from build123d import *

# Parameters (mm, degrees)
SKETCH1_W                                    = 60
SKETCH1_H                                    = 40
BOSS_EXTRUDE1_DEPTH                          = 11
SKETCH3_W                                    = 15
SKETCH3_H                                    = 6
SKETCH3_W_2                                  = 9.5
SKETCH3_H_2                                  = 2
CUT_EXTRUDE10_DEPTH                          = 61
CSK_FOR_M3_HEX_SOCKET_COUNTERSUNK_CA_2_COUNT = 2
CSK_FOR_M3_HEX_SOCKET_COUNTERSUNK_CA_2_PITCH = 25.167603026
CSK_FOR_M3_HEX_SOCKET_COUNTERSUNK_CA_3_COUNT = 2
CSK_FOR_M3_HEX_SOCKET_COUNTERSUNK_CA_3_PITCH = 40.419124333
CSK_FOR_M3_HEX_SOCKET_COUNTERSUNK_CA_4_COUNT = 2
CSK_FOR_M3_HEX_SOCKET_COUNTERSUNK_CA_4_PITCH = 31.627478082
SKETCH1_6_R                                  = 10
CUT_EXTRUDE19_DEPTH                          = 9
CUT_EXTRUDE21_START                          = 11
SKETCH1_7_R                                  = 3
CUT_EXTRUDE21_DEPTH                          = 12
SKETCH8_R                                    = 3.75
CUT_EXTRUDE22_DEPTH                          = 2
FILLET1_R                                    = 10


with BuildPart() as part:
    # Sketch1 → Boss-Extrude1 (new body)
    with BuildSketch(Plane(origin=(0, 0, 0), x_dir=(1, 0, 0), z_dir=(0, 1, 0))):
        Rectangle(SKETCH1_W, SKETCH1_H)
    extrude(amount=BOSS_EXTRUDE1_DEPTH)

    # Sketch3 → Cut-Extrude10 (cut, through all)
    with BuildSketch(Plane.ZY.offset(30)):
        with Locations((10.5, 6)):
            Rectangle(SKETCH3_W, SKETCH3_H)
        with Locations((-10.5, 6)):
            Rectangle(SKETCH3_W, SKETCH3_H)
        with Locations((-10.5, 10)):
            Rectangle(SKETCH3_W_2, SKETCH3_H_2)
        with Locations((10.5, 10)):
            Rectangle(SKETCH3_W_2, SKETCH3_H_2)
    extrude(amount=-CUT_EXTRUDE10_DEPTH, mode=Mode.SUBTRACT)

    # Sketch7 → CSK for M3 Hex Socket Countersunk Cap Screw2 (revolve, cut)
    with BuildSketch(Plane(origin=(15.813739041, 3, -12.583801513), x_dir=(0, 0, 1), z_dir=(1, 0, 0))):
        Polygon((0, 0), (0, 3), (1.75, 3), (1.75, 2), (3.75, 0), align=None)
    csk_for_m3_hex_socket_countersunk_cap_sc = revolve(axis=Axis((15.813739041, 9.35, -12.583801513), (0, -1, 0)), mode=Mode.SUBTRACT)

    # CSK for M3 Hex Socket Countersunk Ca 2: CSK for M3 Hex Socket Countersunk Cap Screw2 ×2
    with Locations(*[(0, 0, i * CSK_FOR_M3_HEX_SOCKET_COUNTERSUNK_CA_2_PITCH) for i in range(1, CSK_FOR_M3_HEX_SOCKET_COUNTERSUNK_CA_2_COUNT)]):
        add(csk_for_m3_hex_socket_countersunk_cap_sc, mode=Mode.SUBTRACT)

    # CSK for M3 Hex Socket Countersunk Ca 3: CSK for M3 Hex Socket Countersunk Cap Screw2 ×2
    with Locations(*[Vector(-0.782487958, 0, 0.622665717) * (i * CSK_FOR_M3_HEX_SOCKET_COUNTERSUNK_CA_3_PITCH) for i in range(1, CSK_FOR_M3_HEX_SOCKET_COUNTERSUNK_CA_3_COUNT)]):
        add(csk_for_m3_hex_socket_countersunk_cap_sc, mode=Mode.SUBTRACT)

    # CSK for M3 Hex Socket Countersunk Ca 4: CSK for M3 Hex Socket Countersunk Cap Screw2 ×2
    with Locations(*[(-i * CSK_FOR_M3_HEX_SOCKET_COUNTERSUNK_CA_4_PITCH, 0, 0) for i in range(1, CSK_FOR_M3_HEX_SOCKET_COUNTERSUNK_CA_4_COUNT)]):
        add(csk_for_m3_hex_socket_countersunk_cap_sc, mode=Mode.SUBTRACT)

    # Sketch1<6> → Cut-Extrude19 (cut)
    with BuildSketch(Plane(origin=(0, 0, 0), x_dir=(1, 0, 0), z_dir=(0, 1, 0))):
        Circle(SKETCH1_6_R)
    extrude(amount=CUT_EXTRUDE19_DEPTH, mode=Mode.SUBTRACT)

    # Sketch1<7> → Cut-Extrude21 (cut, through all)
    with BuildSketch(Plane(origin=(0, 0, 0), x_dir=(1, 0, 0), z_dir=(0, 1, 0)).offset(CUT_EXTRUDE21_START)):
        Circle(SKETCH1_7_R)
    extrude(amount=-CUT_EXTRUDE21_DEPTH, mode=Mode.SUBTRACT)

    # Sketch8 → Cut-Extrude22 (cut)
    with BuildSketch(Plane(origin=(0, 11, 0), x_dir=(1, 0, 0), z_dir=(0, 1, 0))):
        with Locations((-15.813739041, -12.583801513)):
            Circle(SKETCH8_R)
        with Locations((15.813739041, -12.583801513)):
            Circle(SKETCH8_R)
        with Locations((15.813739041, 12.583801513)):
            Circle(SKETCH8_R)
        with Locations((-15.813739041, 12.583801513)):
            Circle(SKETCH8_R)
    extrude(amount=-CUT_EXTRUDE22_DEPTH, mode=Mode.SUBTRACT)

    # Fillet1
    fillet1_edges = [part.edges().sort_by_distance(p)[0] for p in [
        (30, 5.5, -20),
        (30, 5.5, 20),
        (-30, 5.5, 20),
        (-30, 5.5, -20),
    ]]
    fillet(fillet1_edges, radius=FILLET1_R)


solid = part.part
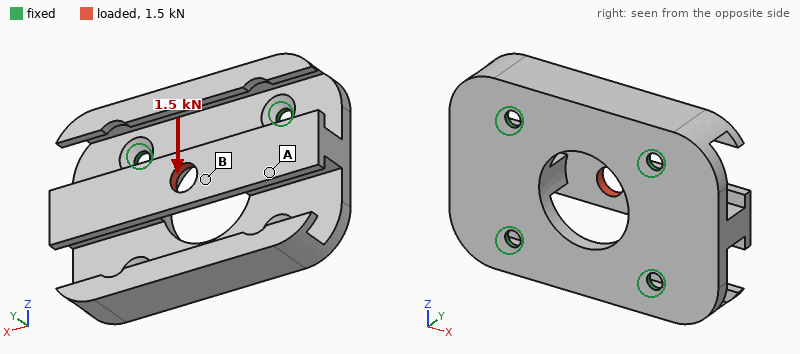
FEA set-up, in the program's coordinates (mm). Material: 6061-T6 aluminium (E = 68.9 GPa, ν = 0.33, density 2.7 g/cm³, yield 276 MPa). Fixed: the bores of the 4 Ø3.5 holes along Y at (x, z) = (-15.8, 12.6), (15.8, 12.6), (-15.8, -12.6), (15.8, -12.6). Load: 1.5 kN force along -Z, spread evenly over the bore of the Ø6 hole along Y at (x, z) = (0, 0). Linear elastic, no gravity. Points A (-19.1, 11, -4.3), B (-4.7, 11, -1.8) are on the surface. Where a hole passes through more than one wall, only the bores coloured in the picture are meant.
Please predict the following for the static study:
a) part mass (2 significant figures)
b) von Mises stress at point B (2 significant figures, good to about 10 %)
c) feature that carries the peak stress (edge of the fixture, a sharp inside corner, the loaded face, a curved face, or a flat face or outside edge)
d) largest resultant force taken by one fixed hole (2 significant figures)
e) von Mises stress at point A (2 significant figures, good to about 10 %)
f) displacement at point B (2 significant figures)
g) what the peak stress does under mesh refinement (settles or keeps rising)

29 g
79 MPa
edge of the fixture
510 N
20 MPa
68 µm
keeps rising
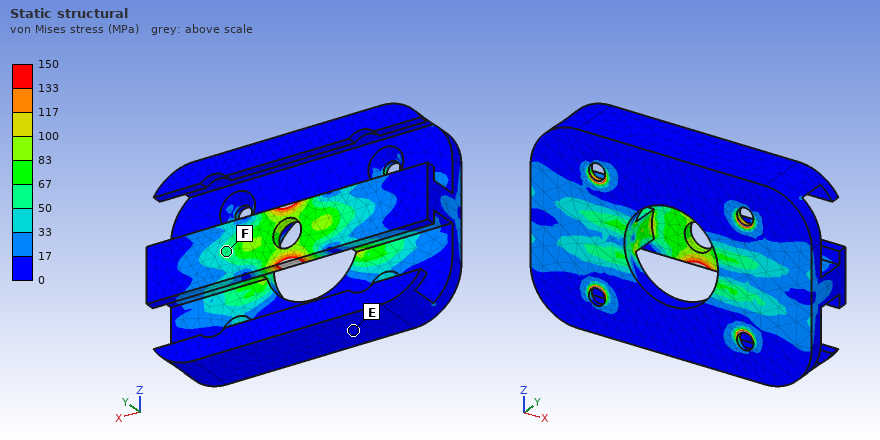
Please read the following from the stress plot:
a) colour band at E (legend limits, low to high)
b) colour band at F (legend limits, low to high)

0 to 17 MPa
50 to 67 MPa
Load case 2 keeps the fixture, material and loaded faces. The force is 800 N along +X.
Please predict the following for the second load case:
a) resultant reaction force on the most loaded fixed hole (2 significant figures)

230 N
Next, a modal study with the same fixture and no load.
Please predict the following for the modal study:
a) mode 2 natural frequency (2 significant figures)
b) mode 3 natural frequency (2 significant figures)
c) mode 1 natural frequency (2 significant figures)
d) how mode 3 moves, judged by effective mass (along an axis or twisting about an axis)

7500 Hz
8100 Hz
7100 Hz
along Z
